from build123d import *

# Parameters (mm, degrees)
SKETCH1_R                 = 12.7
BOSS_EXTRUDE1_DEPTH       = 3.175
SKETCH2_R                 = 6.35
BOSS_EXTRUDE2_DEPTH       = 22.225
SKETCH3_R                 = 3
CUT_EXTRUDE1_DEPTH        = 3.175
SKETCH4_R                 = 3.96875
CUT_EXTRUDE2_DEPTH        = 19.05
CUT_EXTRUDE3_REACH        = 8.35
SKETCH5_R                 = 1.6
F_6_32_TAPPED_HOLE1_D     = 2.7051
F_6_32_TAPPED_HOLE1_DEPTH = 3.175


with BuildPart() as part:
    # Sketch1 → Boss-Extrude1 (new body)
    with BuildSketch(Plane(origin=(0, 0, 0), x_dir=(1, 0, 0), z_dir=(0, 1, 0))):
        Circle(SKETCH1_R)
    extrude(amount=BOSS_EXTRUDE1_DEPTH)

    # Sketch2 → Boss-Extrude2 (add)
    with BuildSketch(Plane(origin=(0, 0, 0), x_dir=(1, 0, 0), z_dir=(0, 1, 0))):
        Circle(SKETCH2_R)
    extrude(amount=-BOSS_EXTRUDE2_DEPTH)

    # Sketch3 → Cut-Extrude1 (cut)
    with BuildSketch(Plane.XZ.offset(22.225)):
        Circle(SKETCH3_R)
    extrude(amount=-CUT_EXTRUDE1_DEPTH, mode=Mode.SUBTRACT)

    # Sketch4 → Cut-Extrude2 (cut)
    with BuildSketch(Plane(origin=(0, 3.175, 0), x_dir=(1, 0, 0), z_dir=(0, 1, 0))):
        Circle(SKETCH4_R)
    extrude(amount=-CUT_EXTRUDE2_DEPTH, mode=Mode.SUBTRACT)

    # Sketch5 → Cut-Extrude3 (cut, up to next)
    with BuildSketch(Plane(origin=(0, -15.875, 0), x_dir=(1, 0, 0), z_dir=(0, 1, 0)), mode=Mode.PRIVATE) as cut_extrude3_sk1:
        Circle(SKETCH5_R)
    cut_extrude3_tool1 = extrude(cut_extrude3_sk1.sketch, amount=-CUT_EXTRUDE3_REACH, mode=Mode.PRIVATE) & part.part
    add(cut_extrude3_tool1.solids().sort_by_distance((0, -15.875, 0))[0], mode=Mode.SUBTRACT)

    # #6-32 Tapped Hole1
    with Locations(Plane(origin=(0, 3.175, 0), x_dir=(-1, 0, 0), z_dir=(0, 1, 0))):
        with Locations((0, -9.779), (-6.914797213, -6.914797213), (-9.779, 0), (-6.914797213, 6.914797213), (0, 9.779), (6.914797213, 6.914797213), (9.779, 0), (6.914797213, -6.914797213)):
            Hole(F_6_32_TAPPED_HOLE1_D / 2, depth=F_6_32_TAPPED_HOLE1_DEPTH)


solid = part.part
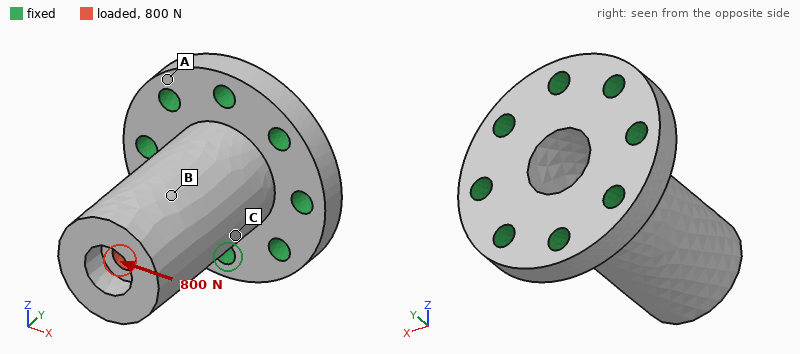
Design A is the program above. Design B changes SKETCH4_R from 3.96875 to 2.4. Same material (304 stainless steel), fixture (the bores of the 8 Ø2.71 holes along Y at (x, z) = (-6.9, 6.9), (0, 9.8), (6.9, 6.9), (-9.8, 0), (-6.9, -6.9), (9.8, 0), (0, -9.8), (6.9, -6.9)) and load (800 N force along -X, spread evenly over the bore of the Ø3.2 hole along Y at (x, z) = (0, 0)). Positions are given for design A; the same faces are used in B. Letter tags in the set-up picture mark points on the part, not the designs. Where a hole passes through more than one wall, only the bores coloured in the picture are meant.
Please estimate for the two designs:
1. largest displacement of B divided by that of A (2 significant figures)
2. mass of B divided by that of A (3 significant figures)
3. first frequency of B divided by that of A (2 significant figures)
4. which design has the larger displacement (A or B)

0.84
1.19
1.0
A
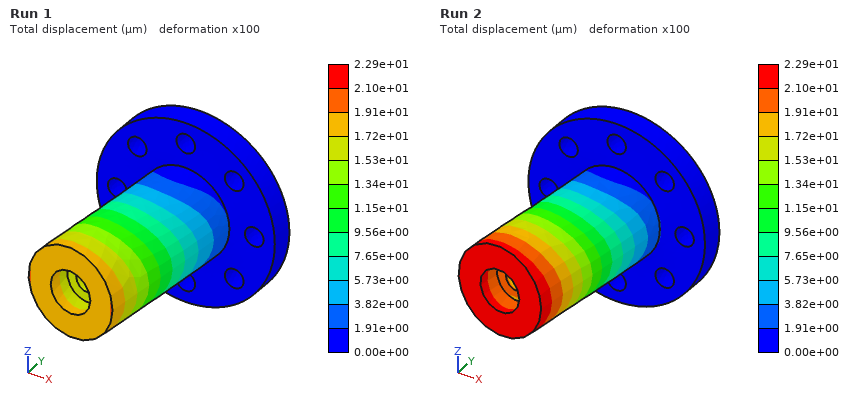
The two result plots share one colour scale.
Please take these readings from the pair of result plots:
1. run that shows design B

Run 1
